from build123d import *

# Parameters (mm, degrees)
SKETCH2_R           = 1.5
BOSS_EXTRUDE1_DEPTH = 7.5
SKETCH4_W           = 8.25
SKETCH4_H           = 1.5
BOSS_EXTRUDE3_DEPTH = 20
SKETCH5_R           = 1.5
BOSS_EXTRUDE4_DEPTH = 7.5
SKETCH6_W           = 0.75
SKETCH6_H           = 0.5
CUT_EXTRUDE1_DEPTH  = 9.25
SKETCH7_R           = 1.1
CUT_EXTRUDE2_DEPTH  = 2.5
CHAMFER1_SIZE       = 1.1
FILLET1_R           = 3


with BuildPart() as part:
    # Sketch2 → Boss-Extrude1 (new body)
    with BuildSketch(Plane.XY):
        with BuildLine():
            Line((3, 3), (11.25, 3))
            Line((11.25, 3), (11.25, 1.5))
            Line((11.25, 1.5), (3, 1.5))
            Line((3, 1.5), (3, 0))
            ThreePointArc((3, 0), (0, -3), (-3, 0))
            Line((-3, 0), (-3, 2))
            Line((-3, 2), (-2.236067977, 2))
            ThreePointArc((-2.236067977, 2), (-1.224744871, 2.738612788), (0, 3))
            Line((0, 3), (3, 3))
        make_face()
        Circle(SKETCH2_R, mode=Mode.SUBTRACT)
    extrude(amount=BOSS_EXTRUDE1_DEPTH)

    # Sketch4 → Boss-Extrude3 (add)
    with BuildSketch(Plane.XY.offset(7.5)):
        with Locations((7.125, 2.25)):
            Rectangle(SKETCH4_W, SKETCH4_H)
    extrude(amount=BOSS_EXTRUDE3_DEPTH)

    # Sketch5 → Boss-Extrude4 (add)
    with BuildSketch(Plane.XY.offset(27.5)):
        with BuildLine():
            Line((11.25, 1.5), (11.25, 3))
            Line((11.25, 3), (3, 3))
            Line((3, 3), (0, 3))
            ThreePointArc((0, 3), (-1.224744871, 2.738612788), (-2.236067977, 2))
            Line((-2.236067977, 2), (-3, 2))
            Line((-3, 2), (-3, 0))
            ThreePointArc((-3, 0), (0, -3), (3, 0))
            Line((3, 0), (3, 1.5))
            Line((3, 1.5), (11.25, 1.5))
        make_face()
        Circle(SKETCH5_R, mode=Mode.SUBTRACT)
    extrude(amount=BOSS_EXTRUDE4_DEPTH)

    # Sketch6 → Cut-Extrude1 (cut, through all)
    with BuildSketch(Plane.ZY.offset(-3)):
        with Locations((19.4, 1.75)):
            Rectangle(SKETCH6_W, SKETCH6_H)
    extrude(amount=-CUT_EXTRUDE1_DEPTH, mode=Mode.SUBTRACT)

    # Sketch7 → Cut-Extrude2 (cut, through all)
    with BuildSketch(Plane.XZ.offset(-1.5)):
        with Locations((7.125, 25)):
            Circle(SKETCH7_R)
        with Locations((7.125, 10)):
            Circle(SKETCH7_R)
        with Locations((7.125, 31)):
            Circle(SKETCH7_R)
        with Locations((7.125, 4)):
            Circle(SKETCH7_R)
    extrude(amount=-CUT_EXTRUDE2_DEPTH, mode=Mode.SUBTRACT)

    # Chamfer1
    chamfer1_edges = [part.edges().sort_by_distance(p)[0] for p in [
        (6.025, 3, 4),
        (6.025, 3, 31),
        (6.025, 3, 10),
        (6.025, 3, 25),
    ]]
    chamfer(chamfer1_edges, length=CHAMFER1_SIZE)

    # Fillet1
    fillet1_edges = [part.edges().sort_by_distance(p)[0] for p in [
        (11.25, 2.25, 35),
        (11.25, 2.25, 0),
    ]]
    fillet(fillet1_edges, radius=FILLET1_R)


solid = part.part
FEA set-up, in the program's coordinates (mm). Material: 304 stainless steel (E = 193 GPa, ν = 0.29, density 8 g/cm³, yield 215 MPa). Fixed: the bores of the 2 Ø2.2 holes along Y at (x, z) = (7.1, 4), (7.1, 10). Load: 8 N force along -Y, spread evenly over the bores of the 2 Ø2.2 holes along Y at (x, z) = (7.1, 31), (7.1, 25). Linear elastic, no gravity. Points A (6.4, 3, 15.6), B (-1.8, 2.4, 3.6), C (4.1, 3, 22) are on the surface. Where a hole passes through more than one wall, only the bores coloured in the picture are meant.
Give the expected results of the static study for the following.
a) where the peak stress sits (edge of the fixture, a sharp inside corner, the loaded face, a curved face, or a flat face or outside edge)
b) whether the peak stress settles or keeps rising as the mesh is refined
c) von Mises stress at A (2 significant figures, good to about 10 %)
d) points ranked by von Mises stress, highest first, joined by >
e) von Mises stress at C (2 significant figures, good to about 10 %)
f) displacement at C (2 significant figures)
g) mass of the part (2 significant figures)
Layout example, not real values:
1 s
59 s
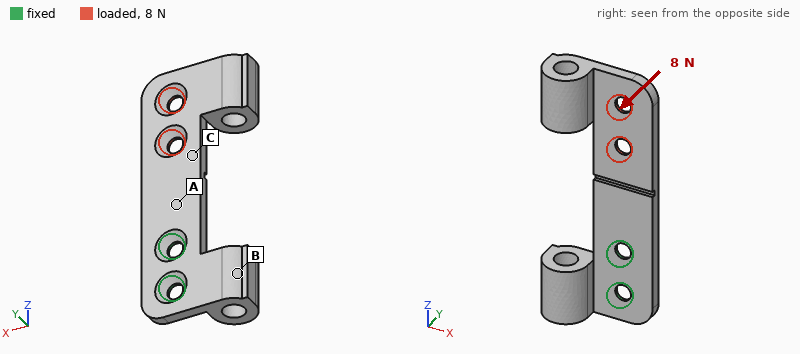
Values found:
edge of the fixture
keeps rising
28 MPa
A > C > B
18 MPa
25 µm
5.9 g
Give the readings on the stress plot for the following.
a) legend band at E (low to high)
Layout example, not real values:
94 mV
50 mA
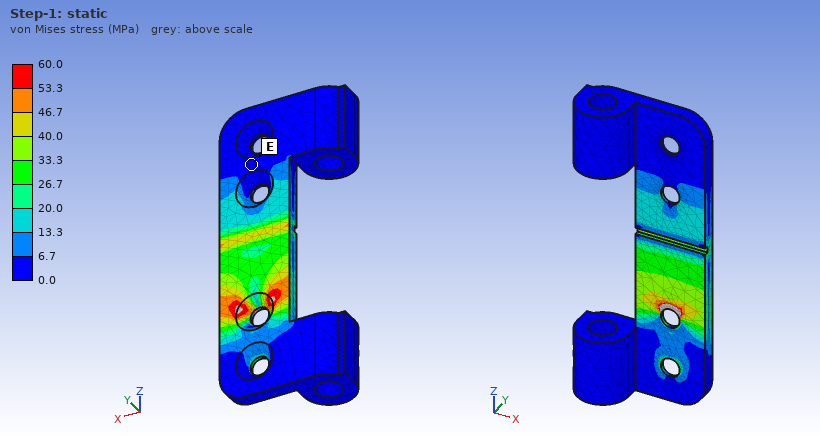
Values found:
0.0 to 6.7 MPa
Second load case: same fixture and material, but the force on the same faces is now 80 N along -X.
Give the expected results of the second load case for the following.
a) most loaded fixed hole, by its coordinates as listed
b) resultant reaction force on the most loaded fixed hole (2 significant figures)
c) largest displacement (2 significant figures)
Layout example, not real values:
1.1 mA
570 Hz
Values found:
(7.1, 10)
240 N
44 µm
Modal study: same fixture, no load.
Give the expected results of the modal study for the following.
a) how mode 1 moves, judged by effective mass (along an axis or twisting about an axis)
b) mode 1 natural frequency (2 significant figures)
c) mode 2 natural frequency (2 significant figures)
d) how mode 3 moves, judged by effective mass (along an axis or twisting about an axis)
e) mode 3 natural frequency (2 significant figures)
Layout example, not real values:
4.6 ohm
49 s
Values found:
along Y
1000 Hz
3500 Hz
along X
5000 Hz
